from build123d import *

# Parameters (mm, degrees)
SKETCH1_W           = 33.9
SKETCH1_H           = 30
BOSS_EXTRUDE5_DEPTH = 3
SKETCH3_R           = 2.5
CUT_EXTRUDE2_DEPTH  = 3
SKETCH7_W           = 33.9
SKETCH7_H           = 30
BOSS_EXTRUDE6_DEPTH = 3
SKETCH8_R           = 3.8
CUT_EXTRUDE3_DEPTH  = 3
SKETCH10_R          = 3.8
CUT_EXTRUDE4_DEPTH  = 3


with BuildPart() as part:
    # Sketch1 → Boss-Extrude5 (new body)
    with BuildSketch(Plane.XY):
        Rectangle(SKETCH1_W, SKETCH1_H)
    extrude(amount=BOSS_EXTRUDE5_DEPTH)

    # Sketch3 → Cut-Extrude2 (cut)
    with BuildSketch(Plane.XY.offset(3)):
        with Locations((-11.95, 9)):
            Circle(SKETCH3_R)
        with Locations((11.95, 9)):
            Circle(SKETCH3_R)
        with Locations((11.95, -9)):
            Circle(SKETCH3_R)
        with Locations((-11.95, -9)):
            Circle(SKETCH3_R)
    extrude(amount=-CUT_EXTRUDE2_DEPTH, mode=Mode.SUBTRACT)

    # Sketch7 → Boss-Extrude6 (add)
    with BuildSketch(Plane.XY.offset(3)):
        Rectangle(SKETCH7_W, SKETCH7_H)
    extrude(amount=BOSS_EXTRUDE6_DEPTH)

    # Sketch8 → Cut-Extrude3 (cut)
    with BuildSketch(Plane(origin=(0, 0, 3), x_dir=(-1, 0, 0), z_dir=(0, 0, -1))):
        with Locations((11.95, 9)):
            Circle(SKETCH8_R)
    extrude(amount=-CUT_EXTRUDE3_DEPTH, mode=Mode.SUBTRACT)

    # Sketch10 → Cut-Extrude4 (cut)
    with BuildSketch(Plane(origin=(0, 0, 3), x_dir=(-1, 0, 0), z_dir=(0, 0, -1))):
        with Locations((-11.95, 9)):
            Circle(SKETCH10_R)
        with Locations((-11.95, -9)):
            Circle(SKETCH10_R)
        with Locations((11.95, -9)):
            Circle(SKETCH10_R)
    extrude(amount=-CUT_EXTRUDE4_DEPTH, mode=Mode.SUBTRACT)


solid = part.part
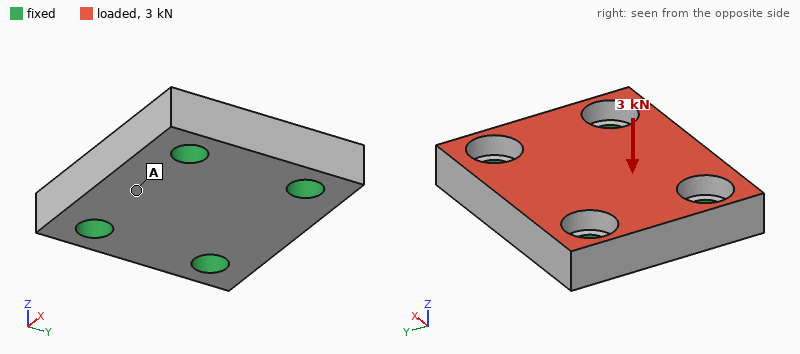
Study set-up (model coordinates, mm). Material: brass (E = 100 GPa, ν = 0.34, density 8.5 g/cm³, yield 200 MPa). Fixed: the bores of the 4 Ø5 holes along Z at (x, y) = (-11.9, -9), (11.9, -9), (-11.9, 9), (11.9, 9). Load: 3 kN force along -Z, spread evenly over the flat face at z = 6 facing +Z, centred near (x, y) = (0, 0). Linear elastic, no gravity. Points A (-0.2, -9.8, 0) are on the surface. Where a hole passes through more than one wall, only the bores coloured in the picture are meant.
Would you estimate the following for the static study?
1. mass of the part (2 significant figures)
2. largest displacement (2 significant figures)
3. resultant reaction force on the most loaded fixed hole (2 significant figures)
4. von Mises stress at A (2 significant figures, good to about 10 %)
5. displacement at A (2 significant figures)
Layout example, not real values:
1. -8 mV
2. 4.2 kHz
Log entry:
1. 45 g
2. 4.0 µm
3. 800 N
4. 14 MPa
5. 3.6 µm
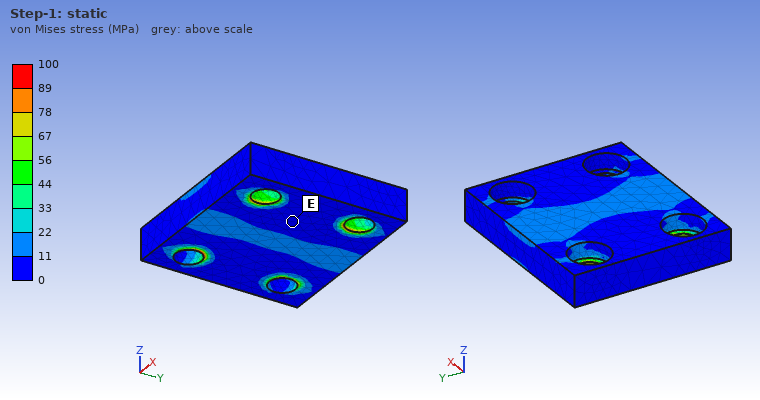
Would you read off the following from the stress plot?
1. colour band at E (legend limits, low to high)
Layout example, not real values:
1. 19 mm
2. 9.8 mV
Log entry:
1. 0 to 11 MPa
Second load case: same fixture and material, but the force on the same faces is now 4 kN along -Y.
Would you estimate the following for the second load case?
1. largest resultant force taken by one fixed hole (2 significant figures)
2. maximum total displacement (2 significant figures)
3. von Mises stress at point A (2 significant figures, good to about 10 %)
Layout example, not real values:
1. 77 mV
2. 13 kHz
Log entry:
1. 1.1 kN
2. 6.1 µm
3. 10 MPa
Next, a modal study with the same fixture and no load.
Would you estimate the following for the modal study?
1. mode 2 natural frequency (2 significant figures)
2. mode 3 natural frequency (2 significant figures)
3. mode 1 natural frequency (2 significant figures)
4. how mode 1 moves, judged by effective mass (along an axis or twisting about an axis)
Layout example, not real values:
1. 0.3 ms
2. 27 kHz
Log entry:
1. 26 kHz
2. 33 kHz
3. 23 kHz
4. along Z
